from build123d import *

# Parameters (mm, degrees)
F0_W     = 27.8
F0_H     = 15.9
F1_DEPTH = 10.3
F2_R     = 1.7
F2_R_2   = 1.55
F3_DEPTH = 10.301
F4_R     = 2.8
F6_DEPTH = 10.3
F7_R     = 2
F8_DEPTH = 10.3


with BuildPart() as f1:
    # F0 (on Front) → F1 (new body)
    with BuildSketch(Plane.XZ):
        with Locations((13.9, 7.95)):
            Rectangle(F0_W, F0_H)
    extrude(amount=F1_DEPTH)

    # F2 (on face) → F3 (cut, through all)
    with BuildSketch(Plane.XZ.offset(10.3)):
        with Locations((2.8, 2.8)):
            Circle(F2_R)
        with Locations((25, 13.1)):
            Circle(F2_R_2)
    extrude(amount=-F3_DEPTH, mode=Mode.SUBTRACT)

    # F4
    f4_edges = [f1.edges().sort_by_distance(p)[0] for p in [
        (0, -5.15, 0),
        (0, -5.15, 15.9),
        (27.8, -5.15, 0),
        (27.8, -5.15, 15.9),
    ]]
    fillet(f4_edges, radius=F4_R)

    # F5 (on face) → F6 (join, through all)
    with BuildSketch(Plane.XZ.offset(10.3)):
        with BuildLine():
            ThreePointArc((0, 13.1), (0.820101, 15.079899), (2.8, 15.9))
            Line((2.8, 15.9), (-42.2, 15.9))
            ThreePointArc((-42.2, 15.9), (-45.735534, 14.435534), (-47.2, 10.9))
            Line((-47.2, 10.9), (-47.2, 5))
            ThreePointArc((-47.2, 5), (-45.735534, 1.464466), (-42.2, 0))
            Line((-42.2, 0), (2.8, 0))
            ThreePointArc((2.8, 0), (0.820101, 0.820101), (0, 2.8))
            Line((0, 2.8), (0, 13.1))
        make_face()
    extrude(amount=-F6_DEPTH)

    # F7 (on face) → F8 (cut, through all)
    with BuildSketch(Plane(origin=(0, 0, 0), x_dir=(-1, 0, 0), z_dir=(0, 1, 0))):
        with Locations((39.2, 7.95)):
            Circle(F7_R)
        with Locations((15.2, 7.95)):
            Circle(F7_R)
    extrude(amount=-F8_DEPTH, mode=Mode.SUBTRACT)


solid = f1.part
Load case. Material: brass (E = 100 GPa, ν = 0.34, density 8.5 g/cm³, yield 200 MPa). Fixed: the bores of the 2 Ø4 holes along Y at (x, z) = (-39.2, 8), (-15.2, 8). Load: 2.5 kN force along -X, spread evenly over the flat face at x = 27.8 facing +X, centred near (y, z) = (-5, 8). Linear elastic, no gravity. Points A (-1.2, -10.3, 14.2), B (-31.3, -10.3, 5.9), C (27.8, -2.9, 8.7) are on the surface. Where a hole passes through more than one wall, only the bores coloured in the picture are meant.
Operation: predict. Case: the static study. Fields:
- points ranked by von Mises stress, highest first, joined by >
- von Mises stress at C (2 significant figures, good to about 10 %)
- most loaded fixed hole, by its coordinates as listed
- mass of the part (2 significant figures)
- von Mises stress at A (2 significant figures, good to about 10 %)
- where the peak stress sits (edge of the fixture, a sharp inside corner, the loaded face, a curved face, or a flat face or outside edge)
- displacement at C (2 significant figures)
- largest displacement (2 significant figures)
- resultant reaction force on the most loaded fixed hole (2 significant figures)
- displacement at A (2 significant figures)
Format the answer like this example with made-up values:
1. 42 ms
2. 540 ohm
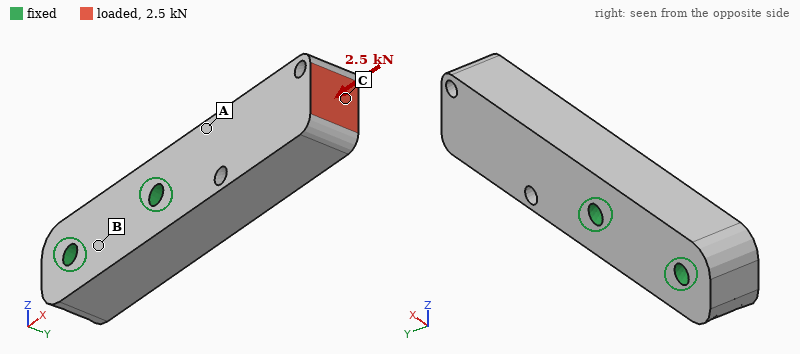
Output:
1. C > A > B
2. 24 MPa
3. (-15.2, 8)
4. 100 g
5. 14 MPa
6. a curved face
7. 8.0 µm
8. 8.4 µm
9. 2.3 kN
10. 2.4 µm
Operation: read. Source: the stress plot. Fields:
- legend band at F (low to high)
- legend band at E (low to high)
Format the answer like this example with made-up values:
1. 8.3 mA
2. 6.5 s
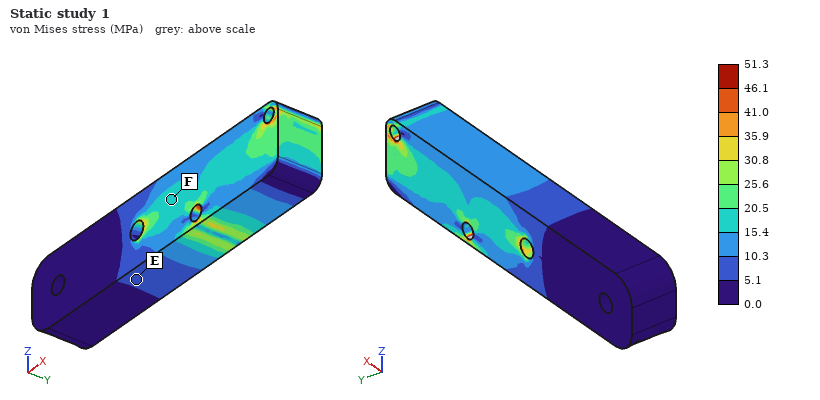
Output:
1. 15.4 to 20.5 MPa
2. 5.1 to 10.3 MPa
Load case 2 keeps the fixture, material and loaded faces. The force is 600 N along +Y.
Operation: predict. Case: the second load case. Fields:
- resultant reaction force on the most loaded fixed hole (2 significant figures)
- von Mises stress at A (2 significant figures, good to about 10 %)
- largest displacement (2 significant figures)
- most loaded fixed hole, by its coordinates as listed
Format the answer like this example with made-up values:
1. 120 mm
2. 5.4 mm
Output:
1. 830 N
2. 66 MPa
3. 0.13 mm
4. (-15.2, 8)
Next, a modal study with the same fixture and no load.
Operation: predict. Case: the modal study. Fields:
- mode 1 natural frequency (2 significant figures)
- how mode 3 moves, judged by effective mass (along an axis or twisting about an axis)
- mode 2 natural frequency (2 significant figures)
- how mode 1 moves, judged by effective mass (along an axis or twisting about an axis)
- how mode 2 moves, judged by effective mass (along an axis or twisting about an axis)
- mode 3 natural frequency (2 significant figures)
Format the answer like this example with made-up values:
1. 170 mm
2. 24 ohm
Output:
1. 2900 Hz
2. twisting about X
3. 3600 Hz
4. along Y
5. along Z
6. 10 kHz
